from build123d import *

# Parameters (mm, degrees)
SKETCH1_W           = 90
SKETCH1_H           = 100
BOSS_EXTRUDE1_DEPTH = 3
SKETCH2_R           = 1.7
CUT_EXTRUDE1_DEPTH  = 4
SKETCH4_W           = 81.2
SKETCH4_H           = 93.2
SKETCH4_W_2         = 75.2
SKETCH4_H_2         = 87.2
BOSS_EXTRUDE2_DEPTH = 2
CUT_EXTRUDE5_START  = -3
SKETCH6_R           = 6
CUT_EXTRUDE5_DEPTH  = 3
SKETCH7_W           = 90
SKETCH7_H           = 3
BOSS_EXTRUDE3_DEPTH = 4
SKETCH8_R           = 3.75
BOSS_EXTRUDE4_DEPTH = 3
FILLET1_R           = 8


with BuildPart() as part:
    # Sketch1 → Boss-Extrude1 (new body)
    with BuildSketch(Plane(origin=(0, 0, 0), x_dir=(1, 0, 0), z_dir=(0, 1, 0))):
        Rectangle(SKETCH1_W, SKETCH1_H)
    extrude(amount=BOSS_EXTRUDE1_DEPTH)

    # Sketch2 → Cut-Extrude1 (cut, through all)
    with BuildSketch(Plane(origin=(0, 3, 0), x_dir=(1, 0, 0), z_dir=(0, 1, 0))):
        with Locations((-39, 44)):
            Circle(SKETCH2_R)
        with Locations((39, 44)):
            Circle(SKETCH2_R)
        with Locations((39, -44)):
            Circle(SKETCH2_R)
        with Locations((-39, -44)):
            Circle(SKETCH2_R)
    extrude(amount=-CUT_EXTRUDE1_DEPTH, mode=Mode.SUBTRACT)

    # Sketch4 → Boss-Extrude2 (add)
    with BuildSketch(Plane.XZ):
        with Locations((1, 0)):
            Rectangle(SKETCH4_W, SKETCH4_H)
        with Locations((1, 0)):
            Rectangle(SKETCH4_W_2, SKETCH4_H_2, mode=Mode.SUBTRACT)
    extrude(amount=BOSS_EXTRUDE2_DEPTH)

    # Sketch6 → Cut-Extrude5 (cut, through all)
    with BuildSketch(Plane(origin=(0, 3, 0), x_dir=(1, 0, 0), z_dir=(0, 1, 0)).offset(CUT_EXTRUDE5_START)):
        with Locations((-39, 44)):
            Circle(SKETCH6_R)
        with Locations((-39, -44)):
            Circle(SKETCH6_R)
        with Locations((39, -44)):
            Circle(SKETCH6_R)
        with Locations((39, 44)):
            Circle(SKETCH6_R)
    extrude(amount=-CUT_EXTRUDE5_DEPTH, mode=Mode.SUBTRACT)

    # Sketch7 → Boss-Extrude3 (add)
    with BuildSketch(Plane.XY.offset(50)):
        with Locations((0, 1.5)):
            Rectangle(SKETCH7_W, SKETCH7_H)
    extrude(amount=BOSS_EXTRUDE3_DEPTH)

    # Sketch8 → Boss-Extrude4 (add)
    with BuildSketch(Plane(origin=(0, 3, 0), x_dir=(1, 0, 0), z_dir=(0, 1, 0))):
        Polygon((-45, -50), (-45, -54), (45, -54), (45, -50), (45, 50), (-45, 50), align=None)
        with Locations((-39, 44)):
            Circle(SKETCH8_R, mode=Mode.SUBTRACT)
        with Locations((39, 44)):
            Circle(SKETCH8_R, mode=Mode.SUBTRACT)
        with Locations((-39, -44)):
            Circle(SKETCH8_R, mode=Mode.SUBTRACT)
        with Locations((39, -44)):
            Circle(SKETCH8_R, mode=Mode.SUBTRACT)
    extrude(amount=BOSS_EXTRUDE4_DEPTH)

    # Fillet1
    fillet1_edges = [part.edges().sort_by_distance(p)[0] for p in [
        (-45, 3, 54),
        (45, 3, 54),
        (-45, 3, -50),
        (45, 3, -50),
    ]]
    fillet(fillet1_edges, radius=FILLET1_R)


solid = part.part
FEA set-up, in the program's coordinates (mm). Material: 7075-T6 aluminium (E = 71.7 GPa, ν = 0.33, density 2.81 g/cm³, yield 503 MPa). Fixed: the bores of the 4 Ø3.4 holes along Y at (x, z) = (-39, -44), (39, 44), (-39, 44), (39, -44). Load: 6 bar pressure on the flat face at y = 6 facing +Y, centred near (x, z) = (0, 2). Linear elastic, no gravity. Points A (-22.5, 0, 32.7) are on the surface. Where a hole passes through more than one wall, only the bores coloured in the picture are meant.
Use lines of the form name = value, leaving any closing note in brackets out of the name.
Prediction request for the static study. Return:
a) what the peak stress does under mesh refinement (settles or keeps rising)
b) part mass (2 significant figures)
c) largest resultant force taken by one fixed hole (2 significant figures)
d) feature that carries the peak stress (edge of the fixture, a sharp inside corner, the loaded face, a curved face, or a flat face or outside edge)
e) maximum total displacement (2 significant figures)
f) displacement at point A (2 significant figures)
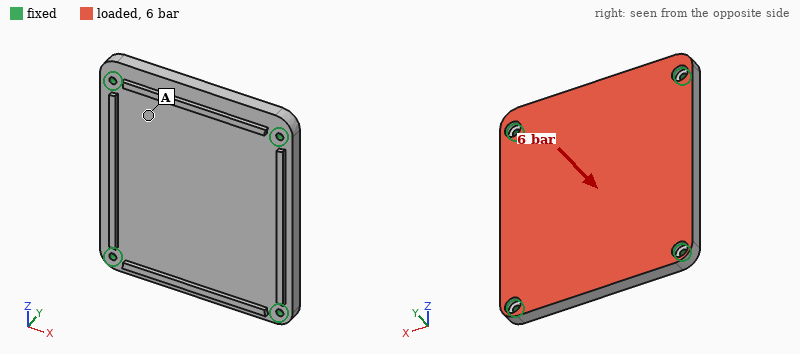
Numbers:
what the peak stress does under mesh refinement = keeps rising
part mass = 160 g
largest resultant force taken by one fixed hole = 2.3 kN
feature that carries the peak stress = edge of the fixture
maximum total displacement = 0.24 mm
displacement at point A = 0.12 mm
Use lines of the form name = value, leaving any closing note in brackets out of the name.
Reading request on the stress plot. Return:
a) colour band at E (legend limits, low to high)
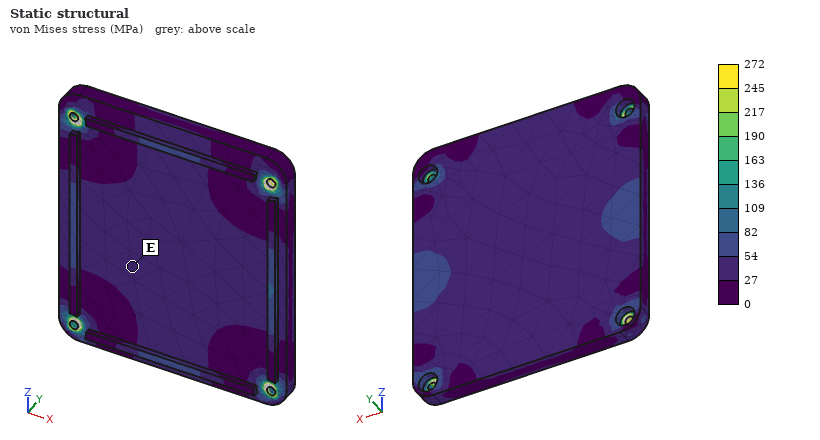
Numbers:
colour band at E = 27 to 54 MPa
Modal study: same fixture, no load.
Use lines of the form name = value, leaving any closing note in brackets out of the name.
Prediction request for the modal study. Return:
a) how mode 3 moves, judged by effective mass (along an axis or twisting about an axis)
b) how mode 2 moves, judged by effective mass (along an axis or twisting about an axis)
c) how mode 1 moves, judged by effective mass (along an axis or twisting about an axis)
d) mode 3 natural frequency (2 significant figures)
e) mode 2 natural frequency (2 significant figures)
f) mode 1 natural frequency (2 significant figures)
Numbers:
how mode 3 moves, judged by effective mass = twisting about X
how mode 2 moves, judged by effective mass = twisting about Z
how mode 1 moves, judged by effective mass = along Y
mode 3 natural frequency = 4100 Hz
mode 2 natural frequency = 3800 Hz
mode 1 natural frequency = 2300 Hz
